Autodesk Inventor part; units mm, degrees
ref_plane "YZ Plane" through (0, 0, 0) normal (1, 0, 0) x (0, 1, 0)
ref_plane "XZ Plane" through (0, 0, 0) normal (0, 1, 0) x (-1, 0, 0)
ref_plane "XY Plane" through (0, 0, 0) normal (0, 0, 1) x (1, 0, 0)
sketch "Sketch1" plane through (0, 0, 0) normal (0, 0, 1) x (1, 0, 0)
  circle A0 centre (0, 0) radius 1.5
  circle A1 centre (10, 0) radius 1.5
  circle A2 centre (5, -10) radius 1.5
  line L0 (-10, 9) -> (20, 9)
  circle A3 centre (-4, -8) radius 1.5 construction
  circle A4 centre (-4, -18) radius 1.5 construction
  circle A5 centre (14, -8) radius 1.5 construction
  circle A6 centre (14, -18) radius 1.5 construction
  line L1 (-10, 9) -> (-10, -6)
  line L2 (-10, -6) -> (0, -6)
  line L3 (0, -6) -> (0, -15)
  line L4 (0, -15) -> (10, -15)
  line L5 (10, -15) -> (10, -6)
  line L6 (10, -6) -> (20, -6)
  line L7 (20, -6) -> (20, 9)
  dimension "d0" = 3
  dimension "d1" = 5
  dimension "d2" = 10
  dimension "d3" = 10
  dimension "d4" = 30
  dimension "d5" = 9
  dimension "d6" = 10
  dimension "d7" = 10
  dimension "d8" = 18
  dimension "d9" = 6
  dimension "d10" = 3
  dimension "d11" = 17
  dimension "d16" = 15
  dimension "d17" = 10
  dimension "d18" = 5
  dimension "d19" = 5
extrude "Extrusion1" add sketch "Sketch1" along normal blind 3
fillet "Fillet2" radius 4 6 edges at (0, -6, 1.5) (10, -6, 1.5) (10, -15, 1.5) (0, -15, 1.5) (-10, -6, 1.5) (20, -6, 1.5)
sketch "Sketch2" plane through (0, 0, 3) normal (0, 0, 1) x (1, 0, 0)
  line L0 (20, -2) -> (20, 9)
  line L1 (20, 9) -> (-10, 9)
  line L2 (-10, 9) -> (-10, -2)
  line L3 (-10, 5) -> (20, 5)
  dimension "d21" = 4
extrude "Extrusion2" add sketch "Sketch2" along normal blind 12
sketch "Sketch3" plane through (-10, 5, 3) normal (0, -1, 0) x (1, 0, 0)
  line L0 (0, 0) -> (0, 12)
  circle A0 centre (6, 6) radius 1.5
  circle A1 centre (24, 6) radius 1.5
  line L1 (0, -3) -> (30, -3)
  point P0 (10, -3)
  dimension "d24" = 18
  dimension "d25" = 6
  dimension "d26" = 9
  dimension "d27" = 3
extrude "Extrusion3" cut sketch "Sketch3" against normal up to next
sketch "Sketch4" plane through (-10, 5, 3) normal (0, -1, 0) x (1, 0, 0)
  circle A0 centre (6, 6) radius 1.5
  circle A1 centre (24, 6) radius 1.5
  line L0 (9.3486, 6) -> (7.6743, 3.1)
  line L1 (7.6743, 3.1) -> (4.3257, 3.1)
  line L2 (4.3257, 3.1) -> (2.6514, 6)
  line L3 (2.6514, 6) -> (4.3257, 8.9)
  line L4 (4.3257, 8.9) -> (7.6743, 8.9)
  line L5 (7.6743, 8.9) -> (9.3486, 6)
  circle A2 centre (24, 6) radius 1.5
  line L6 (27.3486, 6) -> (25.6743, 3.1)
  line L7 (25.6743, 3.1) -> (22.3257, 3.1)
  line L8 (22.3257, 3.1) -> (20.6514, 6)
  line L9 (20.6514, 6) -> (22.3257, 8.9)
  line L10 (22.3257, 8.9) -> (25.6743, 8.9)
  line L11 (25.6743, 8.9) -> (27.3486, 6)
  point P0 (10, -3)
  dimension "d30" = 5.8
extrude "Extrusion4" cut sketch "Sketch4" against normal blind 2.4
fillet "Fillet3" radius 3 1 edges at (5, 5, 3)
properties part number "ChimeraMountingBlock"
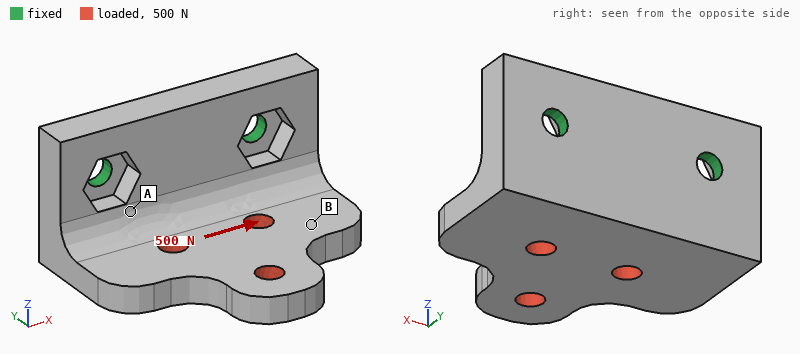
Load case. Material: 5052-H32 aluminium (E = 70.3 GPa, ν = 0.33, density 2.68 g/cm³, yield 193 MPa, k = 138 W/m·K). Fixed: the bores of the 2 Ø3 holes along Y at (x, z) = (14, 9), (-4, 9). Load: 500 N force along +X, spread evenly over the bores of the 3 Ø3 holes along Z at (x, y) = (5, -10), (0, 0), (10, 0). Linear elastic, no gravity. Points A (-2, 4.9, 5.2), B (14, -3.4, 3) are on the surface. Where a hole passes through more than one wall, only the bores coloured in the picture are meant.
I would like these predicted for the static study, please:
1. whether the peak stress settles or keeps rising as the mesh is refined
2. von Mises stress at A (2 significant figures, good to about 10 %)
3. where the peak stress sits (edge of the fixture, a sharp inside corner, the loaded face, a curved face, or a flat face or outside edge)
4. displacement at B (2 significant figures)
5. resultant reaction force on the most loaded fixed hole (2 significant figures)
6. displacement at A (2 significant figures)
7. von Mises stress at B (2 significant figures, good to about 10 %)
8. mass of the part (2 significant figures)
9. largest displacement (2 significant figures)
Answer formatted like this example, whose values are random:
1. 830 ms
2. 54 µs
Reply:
1. keeps rising
2. 37 MPa
3. edge of the fixture
4. 19 µm
5. 440 N
6. 5.3 µm
7. 14 MPa
8. 7.7 g
9. 30 µm
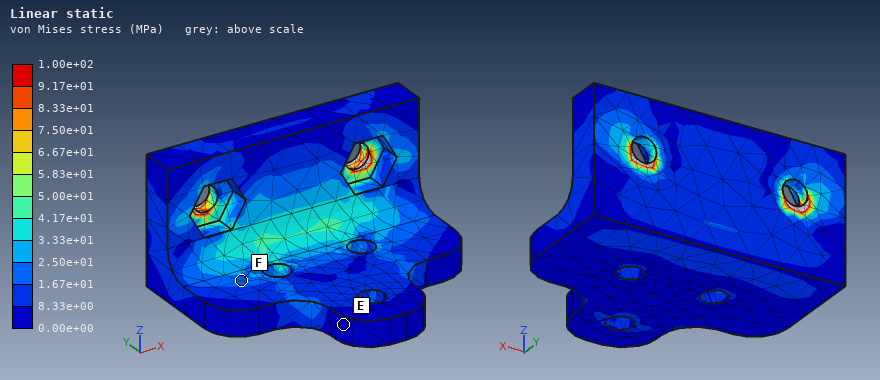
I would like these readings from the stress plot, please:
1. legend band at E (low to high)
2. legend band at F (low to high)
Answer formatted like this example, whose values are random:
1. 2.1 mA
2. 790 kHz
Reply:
1. 0.00e+00 to 8.33e+00 MPa
2. 1.67e+01 to 2.50e+01 MPa
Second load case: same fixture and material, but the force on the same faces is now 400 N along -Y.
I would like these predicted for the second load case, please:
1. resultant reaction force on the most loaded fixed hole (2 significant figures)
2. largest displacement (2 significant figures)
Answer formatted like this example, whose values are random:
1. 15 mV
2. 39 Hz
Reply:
1. 200 N
2. 92 µm
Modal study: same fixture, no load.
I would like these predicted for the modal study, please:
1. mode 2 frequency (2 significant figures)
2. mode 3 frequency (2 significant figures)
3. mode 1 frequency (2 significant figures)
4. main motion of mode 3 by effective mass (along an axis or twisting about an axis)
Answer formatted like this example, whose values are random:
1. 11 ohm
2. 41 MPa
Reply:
1. 12 kHz
2. 14 kHz
3. 4800 Hz
4. along Y
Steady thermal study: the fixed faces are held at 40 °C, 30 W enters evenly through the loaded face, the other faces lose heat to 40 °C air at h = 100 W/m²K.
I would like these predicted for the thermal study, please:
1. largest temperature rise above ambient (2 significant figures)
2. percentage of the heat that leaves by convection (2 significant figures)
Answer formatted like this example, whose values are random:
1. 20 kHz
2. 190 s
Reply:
1. 53 K
2. 15 %
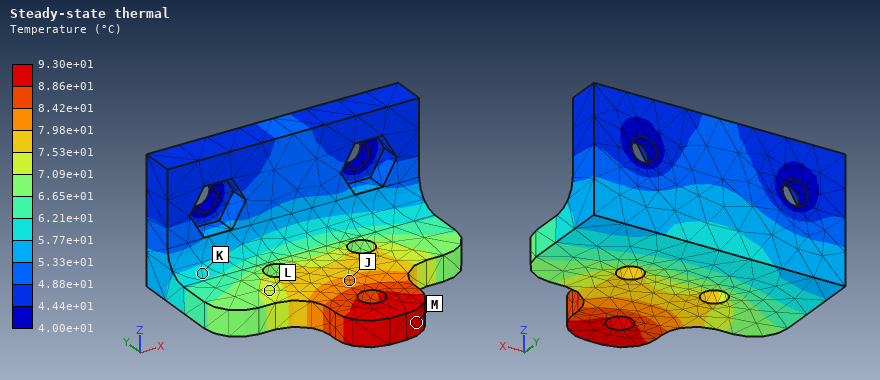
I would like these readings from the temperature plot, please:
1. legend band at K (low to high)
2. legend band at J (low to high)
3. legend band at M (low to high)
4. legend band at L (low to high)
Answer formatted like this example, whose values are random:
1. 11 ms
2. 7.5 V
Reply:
1. 5.77e+01 to 6.21e+01 °C
2. 7.98e+01 to 8.42e+01 °C
3. 8.86e+01 to 9.30e+01 °C
4. 7.09e+01 to 7.53e+01 °C
